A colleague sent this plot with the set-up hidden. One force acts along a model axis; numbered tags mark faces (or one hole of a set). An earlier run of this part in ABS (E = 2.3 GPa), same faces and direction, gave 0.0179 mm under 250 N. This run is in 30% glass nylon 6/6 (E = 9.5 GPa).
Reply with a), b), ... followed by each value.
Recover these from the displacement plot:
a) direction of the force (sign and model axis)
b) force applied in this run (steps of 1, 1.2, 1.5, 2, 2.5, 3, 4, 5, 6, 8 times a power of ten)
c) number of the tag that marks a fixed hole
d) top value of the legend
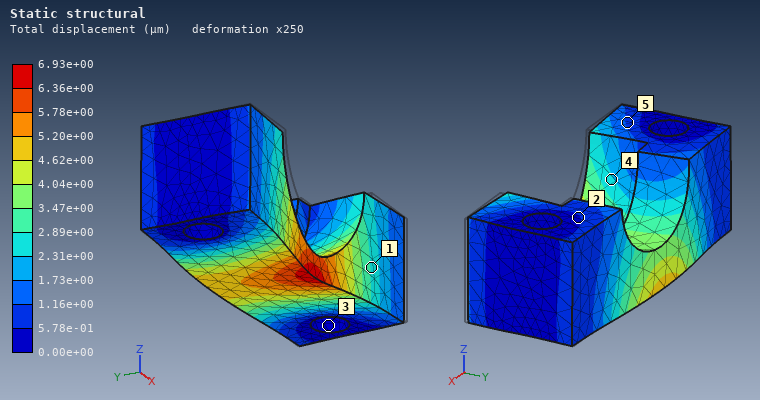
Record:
a) +Y
b) 400 N
c) 3
d) 6.93e+00 µm
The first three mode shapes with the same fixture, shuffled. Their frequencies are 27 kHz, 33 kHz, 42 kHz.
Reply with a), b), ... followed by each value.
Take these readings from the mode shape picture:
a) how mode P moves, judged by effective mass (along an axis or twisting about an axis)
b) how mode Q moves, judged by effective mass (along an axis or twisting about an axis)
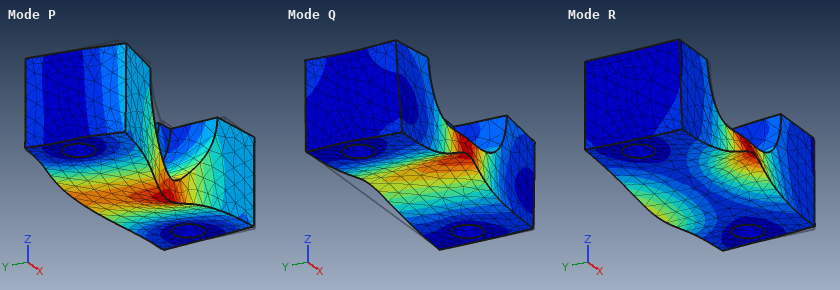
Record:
a) along Y
b) along Z
